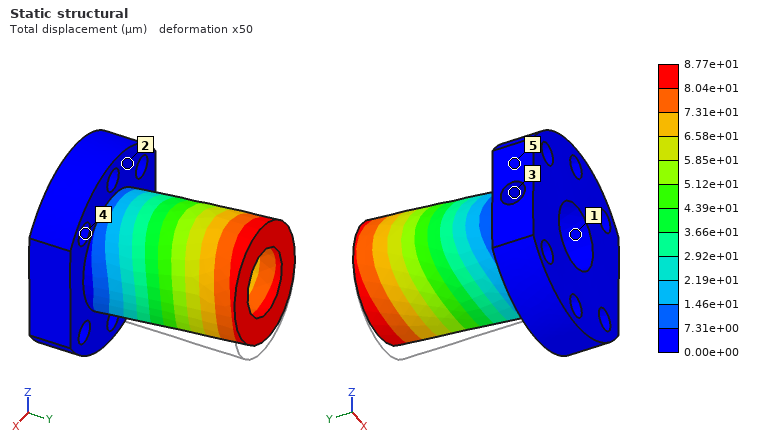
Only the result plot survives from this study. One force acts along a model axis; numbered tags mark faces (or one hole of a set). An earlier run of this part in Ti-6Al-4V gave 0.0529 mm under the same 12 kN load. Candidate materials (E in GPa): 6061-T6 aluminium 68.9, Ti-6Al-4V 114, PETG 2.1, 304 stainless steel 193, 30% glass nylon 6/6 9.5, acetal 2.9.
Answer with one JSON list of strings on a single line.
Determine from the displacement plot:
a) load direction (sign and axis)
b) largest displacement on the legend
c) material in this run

["+Z", "8.77e+01 µm", "6061-T6 aluminium"]
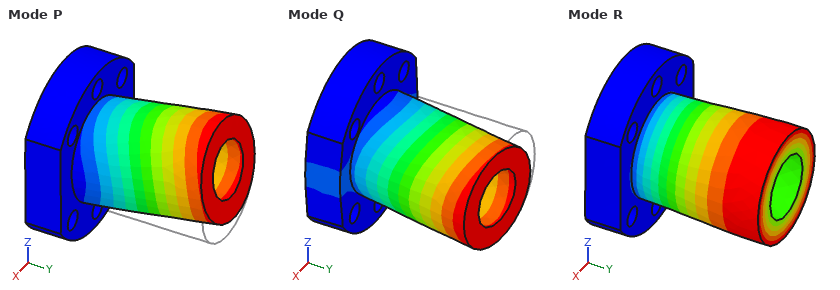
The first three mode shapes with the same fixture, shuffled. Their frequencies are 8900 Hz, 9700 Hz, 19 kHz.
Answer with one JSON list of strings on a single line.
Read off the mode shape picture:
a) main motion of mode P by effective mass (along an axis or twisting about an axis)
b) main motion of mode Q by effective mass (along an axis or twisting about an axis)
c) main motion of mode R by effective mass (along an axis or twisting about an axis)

["along Z", "along X", "twisting about Y"]
